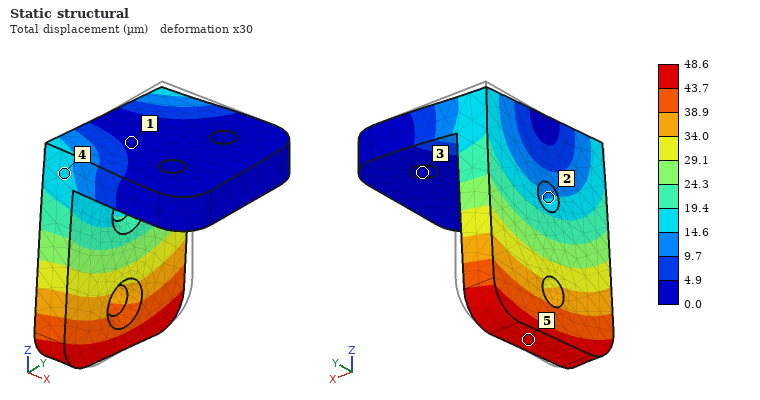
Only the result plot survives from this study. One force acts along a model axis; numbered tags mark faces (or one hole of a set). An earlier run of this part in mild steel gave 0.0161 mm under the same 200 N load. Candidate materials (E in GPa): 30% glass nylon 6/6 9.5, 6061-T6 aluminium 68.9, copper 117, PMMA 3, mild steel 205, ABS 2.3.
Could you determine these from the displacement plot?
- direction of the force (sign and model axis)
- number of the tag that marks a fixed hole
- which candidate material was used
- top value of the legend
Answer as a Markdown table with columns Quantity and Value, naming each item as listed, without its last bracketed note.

| Quantity | Value |
|---|---|
| direction of the force | -Y |
| number of the tag that marks a fixed hole | 3 |
| which candidate material was used | 6061-T6 aluminium |
| top value of the legend | 48.6 µm |
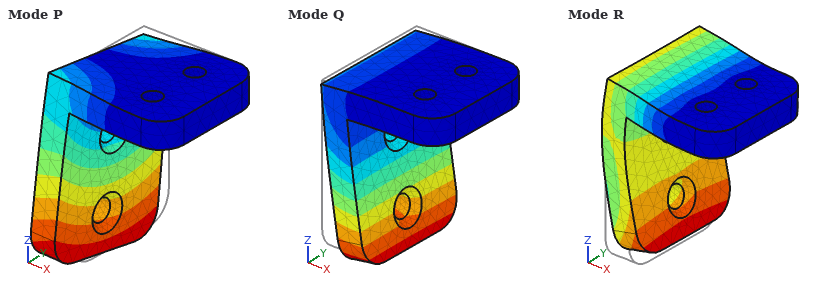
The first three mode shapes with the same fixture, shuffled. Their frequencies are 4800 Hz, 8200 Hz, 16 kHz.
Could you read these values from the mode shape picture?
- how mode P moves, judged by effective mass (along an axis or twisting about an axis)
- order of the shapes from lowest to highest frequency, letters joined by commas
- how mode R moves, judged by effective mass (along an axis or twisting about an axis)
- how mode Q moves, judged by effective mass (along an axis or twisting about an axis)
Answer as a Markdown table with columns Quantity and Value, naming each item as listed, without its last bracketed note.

| Quantity | Value |
|---|---|
| how mode P moves, judged by effective mass | along Y |
| order of the shapes from lowest to highest frequency, letters joined by commas | Q, P, R |
| how mode R moves, judged by effective mass | along Z |
| how mode Q moves, judged by effective mass | along X |
